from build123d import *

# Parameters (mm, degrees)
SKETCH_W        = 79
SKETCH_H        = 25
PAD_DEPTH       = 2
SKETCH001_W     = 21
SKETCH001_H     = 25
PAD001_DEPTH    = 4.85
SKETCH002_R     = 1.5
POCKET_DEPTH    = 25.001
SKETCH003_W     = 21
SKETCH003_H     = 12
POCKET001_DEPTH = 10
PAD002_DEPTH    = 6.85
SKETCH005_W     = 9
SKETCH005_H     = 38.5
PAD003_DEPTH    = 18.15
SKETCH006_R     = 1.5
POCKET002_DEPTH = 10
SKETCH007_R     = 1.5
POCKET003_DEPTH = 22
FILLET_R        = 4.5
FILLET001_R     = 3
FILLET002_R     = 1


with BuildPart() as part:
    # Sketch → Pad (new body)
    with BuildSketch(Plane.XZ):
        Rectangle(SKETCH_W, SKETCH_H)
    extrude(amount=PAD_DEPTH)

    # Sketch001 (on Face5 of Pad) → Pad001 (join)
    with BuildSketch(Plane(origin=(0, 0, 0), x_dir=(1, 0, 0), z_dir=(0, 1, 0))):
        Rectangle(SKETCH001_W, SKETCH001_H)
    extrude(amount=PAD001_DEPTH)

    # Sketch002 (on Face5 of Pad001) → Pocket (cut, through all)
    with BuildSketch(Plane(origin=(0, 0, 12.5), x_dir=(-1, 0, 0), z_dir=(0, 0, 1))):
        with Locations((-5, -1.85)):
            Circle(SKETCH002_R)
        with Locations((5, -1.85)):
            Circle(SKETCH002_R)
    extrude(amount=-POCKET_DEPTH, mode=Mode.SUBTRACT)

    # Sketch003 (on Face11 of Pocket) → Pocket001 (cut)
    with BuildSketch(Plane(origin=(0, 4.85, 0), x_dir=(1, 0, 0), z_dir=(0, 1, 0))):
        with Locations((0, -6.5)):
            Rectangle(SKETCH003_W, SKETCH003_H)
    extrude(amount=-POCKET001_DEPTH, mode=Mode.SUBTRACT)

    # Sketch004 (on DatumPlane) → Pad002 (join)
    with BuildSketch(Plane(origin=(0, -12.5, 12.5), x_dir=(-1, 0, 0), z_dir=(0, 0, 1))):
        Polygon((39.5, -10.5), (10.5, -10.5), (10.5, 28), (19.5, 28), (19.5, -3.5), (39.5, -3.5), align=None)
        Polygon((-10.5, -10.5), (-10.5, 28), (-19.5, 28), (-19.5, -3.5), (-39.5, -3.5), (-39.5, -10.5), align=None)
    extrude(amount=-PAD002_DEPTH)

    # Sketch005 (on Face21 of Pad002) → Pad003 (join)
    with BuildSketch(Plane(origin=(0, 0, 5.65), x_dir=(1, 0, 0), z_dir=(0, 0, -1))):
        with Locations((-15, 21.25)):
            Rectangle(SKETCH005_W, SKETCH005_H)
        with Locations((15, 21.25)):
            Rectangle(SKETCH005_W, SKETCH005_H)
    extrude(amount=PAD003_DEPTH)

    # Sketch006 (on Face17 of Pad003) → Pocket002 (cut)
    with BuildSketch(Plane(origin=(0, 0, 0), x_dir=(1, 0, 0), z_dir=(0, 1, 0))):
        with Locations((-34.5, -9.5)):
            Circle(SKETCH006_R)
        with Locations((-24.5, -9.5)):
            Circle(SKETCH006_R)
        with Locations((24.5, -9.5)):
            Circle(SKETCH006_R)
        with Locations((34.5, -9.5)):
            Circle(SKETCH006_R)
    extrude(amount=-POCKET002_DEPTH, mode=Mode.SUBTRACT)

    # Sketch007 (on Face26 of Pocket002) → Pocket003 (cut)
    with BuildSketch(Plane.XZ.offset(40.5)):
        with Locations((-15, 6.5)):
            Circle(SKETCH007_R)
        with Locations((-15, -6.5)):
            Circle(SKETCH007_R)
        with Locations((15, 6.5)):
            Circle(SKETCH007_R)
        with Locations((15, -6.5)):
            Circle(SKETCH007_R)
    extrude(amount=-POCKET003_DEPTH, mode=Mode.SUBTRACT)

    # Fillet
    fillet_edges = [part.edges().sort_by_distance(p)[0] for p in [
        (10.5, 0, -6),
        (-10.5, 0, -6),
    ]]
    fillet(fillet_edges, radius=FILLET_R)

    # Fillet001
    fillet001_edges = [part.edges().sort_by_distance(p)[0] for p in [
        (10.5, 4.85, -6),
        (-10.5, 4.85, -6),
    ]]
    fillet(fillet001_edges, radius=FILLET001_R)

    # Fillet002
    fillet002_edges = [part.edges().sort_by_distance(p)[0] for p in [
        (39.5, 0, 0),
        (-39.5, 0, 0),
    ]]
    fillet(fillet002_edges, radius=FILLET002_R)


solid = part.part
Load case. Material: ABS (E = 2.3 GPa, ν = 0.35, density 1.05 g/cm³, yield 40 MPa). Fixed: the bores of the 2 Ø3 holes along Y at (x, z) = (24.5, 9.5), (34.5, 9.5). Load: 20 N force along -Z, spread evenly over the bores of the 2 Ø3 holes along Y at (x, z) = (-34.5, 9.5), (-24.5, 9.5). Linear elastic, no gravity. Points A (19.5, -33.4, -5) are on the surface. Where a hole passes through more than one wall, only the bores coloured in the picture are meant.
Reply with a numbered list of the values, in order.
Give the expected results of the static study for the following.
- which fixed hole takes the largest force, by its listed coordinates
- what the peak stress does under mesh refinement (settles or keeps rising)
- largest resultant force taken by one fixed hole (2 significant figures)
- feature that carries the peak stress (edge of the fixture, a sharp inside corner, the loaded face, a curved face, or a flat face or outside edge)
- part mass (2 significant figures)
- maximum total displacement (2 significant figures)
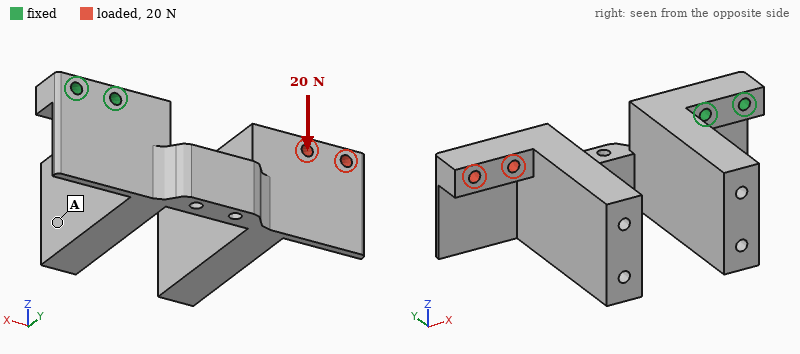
1. (24.5, 9.5)
2. keeps rising
3. 94 N
4. a sharp inside corner
5. 24 g
6. 0.92 mm
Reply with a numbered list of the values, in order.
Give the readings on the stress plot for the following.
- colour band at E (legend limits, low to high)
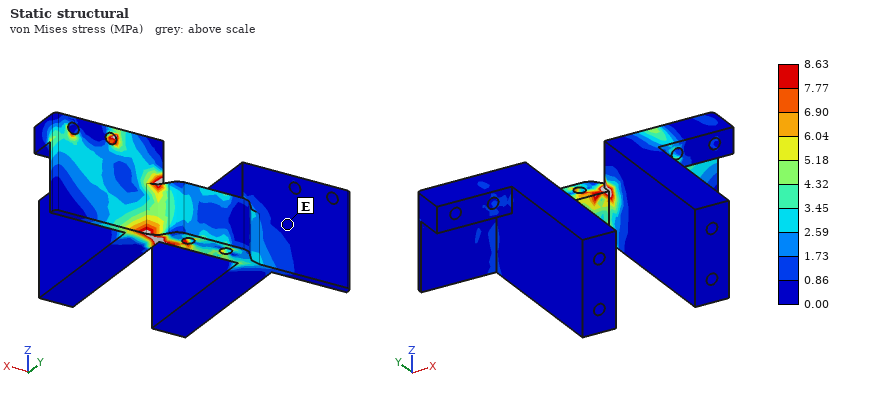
1. 0.00 to 0.86 MPa
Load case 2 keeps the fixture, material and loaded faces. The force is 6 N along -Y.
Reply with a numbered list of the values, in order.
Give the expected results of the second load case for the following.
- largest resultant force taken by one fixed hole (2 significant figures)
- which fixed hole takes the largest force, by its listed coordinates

1. 9.8 N
2. (24.5, 9.5)
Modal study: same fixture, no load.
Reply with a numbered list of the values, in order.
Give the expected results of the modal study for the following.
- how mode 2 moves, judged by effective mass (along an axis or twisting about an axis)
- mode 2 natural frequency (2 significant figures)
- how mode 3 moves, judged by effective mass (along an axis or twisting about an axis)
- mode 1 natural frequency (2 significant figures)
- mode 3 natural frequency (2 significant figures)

1. along Z
2. 240 Hz
3. along Y
4. 160 Hz
5. 460 Hz
